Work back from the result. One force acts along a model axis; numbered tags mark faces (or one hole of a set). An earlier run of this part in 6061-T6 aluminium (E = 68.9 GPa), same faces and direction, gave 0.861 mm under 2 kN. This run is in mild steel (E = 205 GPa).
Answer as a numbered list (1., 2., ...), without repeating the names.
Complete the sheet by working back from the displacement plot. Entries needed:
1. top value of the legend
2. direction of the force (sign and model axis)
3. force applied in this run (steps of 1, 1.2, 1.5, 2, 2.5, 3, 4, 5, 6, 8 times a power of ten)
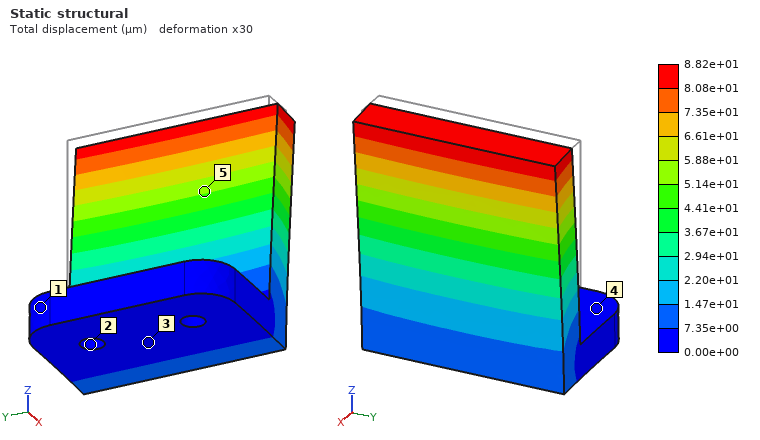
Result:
1. 8.82e+01 µm
2. +X
3. 600 N
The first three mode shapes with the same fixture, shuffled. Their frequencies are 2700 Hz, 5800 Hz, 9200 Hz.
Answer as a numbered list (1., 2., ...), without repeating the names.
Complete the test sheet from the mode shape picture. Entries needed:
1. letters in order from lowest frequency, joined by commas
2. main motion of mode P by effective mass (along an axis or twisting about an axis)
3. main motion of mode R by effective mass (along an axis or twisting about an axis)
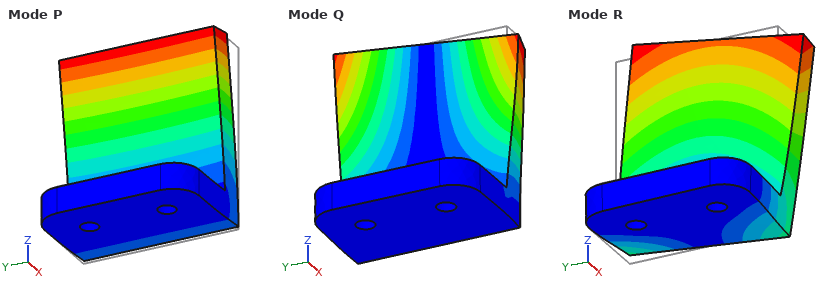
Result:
1. P, R, Q
2. along X
3. along Y
